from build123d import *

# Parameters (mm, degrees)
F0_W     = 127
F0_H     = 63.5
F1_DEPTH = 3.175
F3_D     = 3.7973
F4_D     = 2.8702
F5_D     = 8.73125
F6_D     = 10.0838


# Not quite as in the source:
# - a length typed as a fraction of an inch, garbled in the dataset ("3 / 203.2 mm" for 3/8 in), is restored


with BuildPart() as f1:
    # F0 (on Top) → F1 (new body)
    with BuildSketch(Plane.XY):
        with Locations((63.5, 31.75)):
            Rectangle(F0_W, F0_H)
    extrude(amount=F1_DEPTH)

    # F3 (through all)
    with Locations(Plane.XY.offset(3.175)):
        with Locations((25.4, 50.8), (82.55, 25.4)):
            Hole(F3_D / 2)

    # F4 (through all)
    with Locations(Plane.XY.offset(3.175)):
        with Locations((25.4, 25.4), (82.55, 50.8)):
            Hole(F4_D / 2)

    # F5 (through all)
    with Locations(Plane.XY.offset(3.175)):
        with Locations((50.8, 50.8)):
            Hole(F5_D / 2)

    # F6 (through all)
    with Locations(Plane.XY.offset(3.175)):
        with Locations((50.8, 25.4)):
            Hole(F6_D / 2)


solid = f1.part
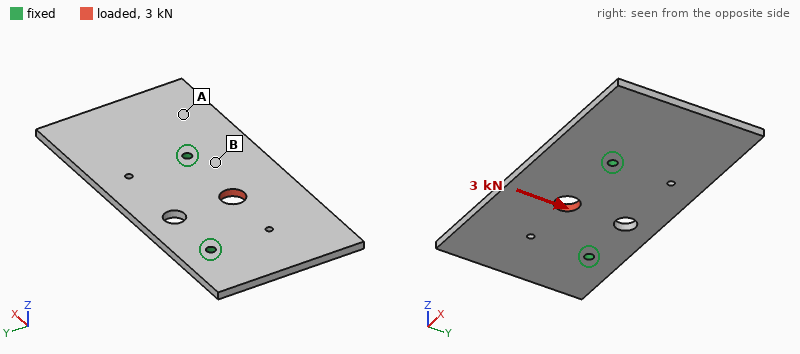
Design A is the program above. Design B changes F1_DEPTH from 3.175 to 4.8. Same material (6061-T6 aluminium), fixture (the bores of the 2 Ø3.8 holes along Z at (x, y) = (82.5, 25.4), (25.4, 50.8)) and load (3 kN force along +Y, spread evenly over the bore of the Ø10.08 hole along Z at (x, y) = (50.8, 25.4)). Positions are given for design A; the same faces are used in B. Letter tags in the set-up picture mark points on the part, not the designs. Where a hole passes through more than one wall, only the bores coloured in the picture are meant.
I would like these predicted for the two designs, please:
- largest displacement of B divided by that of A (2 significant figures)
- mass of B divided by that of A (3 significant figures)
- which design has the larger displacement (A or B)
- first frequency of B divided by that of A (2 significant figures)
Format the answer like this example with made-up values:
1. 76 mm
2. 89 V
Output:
1. 0.66
2. 1.51
3. A
4. 1.4
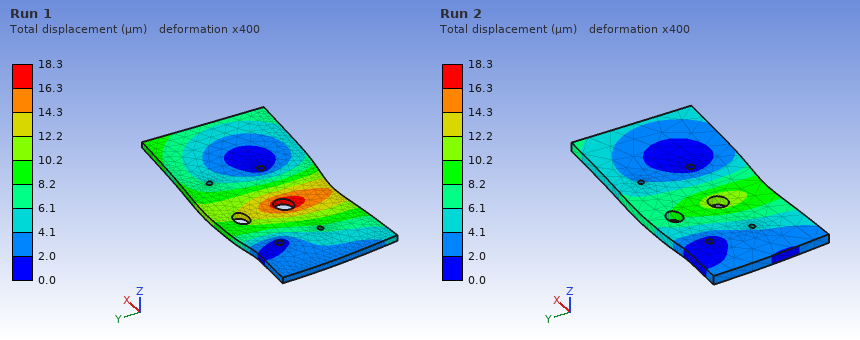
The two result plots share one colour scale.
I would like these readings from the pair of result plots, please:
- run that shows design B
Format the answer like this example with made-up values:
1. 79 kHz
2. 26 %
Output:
1. Run 2
